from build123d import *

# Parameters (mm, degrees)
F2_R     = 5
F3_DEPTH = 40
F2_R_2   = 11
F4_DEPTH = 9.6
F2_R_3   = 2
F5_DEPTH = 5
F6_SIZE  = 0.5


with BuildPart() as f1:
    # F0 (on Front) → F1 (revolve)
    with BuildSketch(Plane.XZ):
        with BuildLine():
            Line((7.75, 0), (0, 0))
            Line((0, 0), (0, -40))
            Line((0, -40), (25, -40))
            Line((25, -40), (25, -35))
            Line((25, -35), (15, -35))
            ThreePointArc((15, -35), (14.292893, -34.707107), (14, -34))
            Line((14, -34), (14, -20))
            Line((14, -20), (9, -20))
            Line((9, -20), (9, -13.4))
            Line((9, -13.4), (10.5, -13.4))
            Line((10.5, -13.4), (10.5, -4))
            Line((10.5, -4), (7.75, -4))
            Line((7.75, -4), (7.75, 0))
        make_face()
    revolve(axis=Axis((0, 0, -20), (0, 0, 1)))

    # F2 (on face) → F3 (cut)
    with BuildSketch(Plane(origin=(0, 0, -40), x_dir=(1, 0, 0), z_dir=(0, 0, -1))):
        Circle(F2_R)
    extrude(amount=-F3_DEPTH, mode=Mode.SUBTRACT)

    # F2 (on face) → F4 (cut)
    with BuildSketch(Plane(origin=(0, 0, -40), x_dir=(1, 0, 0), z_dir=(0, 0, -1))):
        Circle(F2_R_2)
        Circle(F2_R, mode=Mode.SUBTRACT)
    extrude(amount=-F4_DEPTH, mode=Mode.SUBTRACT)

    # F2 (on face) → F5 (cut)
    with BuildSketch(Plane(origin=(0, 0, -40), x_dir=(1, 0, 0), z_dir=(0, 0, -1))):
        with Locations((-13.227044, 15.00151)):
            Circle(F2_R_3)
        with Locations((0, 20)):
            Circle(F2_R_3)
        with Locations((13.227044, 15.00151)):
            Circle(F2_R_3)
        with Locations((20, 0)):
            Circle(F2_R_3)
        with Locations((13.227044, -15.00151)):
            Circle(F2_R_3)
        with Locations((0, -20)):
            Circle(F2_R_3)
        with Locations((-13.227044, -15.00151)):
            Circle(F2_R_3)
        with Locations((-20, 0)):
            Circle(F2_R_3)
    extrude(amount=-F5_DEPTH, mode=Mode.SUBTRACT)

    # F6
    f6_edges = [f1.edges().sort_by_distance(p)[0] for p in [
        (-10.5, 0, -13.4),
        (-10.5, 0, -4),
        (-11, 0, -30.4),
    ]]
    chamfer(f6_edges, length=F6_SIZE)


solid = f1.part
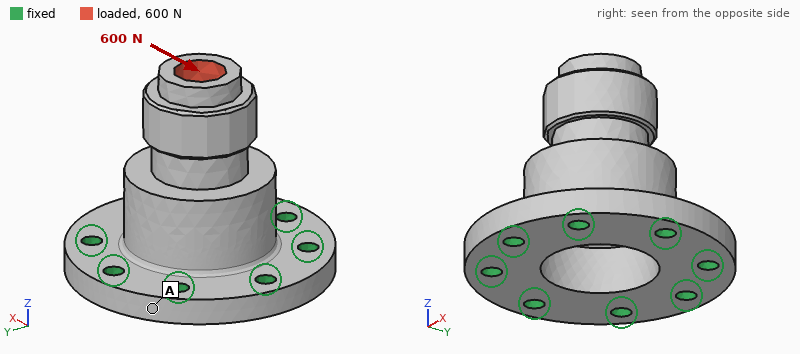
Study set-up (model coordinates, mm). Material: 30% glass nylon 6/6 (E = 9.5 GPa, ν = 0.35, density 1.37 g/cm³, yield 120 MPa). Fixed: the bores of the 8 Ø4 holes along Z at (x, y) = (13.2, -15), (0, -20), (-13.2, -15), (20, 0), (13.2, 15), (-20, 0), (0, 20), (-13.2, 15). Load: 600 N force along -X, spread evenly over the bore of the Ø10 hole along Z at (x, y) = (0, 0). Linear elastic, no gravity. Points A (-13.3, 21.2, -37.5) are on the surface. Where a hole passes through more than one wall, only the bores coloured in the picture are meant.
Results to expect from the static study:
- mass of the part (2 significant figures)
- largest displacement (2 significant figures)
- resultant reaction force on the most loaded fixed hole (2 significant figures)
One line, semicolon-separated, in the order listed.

25 g; 78 µm; 260 N
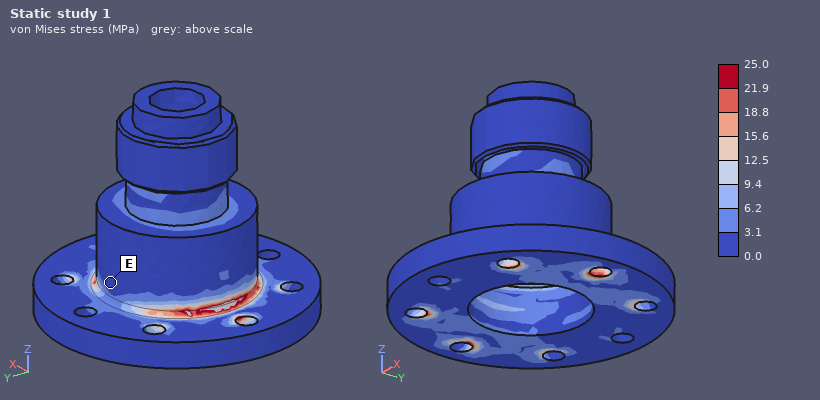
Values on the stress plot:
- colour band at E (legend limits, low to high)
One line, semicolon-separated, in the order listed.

0.0 to 3.1 MPa
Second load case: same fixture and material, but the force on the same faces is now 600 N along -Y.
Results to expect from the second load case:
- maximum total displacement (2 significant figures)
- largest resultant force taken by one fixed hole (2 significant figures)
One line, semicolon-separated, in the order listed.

75 µm; 220 N
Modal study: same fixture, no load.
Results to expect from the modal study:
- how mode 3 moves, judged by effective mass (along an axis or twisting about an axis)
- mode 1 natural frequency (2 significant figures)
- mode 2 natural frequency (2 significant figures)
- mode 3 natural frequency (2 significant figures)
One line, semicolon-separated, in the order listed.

along Z; 5500 Hz; 5600 Hz; 11 kHz
